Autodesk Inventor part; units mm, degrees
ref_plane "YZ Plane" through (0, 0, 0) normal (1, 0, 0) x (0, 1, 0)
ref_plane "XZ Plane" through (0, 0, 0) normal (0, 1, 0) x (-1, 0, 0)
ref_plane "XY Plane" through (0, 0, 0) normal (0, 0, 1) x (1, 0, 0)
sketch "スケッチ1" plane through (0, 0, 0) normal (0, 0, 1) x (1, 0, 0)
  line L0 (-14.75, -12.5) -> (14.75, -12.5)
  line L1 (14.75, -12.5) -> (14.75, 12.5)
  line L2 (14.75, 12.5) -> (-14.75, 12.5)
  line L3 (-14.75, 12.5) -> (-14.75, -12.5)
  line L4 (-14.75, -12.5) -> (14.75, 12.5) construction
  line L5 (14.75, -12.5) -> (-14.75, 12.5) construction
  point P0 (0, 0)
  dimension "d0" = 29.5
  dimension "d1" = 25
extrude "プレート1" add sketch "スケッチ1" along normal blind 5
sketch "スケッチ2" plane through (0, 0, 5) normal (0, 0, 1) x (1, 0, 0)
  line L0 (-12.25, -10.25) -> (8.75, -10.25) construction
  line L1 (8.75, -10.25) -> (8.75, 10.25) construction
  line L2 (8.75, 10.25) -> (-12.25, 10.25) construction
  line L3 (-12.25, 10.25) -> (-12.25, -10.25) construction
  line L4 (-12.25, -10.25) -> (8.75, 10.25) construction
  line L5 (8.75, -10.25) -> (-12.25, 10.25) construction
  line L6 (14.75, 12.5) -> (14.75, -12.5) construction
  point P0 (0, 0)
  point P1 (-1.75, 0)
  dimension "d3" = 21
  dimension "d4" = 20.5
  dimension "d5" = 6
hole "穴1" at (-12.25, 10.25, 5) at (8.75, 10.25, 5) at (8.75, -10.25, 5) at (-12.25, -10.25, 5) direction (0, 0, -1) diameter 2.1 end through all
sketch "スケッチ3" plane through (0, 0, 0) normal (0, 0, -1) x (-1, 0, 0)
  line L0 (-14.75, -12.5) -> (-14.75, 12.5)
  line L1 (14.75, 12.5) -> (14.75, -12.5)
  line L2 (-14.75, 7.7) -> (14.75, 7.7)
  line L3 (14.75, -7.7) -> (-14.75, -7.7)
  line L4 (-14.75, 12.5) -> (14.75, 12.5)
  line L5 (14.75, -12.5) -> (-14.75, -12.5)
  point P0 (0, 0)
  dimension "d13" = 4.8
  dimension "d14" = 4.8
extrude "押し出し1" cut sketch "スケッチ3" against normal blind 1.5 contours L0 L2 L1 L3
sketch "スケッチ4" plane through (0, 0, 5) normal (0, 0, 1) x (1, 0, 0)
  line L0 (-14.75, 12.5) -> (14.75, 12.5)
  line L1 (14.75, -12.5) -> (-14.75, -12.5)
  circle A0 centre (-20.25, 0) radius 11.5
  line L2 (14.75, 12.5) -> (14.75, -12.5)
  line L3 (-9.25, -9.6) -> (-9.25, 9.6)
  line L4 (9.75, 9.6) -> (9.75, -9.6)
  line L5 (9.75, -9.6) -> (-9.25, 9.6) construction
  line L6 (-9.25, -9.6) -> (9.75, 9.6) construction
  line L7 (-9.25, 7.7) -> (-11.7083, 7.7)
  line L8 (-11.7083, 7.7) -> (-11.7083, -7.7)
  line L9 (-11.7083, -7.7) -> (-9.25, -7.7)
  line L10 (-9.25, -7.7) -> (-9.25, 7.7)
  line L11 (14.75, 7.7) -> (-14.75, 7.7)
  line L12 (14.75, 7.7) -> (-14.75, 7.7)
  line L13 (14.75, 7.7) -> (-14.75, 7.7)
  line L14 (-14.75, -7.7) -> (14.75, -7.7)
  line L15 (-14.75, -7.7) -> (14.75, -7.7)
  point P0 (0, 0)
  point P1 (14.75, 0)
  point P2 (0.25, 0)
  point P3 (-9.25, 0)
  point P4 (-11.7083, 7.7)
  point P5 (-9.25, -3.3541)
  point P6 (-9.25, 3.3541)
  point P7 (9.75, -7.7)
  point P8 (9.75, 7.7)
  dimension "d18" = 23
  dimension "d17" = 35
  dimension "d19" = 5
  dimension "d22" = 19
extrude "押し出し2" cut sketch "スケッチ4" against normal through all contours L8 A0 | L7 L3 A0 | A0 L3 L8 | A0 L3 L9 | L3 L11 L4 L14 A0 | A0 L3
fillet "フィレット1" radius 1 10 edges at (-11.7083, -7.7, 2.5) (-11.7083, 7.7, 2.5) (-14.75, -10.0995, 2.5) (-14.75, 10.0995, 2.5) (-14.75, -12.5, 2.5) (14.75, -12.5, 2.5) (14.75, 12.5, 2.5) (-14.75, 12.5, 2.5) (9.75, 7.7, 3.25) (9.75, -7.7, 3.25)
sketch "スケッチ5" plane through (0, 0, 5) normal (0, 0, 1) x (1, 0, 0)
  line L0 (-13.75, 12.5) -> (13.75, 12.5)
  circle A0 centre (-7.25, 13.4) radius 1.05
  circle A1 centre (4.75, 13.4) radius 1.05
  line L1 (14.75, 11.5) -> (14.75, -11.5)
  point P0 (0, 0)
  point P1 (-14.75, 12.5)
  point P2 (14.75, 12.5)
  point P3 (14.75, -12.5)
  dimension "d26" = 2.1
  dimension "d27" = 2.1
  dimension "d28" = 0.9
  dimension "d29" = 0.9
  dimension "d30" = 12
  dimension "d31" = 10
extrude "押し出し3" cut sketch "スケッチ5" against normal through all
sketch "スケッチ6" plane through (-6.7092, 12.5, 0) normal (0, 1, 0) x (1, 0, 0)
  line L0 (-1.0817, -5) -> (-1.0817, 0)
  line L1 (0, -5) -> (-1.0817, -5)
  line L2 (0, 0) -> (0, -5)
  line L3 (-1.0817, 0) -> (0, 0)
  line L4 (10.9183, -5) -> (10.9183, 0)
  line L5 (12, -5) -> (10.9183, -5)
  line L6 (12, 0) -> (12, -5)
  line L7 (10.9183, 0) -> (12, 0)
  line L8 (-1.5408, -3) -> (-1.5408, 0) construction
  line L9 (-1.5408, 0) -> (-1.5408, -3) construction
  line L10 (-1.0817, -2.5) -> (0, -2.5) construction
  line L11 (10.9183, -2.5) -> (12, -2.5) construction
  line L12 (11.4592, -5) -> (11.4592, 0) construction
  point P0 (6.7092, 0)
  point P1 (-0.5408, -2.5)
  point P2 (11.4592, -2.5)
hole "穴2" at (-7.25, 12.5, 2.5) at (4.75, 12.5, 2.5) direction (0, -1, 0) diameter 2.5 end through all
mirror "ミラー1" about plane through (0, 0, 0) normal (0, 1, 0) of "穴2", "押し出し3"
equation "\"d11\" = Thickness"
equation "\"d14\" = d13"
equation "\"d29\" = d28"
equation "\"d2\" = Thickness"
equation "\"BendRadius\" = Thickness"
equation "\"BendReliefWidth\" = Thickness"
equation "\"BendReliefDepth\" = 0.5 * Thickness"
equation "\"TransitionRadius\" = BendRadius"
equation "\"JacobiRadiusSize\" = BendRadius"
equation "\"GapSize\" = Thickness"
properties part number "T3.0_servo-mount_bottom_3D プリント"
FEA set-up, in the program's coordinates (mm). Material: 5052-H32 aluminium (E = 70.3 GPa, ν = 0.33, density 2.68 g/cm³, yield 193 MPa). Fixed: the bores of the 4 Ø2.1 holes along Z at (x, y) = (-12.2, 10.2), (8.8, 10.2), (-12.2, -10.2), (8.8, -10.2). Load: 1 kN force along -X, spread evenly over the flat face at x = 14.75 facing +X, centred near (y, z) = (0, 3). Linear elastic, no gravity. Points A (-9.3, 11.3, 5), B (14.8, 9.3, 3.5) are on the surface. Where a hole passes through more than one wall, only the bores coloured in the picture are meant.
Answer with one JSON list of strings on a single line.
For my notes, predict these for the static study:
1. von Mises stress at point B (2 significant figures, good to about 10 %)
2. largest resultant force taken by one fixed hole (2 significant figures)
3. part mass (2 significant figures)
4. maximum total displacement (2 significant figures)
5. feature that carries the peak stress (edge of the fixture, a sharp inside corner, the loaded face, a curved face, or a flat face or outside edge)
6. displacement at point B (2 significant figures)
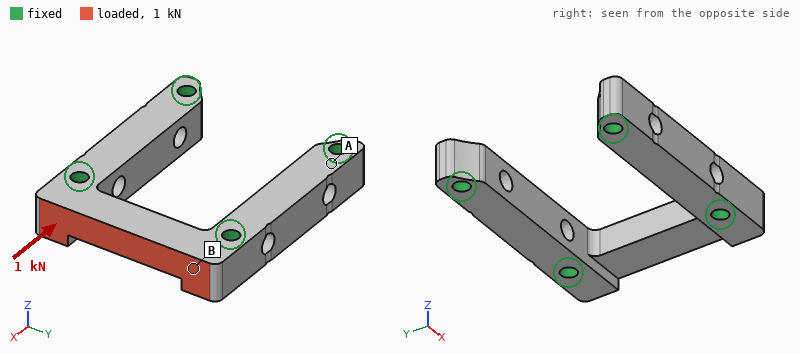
["17 MPa", "550 N", "4.0 g", "10 µm", "a curved face", "3.4 µm"]
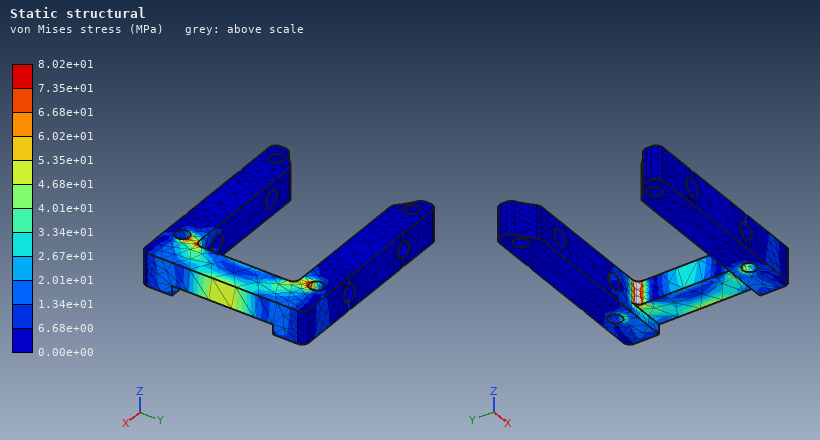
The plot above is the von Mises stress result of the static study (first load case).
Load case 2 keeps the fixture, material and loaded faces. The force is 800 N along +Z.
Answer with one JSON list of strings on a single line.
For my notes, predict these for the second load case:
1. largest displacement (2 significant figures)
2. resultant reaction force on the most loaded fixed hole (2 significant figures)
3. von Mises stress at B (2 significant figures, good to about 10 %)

["29 µm", "410 N", "32 MPa"]
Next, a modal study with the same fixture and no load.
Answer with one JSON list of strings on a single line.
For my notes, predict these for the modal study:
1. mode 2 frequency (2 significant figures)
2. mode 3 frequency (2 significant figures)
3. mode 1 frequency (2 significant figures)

["40 kHz", "40 kHz", "38 kHz"]
